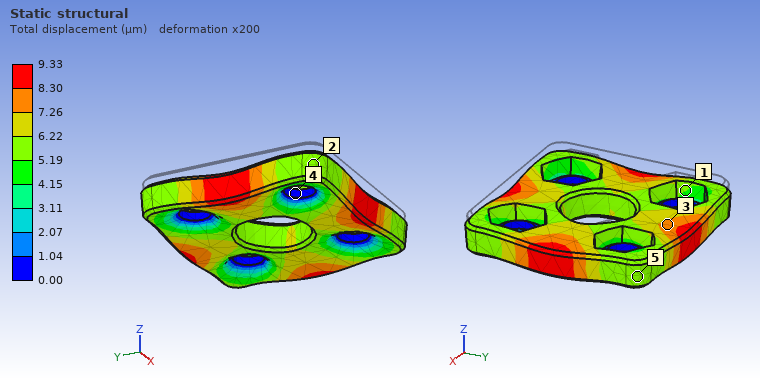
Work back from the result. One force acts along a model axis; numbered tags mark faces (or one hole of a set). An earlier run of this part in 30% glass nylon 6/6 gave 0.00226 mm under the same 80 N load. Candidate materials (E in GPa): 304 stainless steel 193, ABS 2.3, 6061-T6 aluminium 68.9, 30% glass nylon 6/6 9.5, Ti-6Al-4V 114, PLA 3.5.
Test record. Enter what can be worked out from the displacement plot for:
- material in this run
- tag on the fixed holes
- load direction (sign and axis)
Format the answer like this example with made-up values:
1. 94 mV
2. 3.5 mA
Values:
1. ABS
2. 4
3. -Z
